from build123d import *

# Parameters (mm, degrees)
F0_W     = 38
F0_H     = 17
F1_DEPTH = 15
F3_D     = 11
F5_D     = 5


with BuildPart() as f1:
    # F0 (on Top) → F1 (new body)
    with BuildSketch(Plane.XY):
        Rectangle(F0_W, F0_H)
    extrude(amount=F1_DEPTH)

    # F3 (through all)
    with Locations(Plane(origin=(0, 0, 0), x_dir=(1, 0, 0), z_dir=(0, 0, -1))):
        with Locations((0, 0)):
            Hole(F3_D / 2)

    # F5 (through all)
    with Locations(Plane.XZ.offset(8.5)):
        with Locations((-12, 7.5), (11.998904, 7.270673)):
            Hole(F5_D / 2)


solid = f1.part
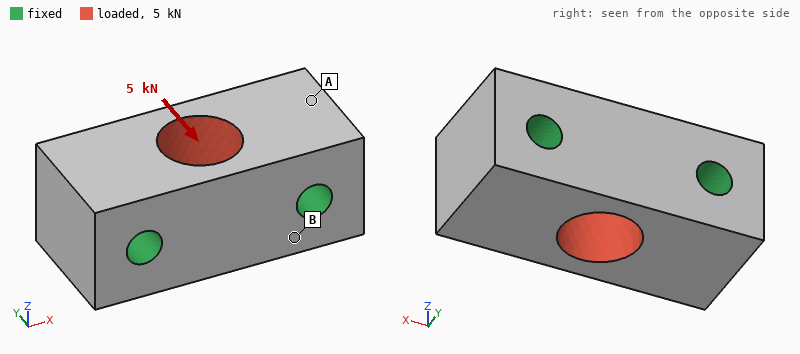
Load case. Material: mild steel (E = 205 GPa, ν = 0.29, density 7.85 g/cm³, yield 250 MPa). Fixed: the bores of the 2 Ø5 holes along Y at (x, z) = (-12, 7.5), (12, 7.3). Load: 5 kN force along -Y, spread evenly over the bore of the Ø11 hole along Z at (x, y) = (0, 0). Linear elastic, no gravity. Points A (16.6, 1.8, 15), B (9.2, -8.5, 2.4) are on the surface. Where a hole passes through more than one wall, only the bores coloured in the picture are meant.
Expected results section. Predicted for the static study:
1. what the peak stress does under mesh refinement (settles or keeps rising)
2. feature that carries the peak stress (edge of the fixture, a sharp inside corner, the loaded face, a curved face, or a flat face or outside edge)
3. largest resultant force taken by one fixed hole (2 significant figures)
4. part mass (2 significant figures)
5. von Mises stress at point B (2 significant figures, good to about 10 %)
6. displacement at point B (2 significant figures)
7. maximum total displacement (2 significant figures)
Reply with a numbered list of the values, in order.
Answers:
1. keeps rising
2. edge of the fixture
3. 2.5 kN
4. 60 g
5. 10 MPa
6. 0.52 µm
7. 2.2 µm
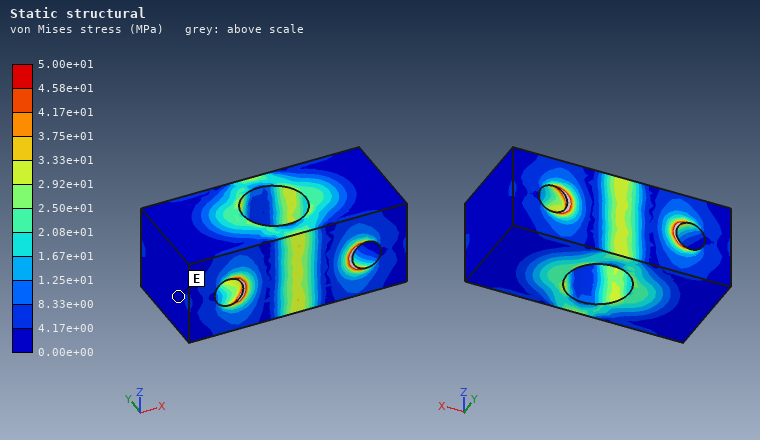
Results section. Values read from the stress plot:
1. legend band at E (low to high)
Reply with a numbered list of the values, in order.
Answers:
1. 0.00e+00 to 4.17e+00 MPa
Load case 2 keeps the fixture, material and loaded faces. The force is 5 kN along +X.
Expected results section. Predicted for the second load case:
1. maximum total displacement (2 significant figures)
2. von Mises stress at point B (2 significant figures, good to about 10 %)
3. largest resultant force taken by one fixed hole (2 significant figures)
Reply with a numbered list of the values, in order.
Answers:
1. 0.65 µm
2. 6.3 MPa
3. 2.5 kN
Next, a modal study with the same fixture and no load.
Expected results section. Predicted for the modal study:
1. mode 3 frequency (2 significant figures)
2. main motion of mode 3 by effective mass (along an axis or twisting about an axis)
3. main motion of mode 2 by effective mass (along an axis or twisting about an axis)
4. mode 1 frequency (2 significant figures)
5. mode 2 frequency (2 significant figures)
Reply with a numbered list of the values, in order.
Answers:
1. 71 kHz
2. along Y
3. twisting about X
4. 56 kHz
5. 67 kHz
